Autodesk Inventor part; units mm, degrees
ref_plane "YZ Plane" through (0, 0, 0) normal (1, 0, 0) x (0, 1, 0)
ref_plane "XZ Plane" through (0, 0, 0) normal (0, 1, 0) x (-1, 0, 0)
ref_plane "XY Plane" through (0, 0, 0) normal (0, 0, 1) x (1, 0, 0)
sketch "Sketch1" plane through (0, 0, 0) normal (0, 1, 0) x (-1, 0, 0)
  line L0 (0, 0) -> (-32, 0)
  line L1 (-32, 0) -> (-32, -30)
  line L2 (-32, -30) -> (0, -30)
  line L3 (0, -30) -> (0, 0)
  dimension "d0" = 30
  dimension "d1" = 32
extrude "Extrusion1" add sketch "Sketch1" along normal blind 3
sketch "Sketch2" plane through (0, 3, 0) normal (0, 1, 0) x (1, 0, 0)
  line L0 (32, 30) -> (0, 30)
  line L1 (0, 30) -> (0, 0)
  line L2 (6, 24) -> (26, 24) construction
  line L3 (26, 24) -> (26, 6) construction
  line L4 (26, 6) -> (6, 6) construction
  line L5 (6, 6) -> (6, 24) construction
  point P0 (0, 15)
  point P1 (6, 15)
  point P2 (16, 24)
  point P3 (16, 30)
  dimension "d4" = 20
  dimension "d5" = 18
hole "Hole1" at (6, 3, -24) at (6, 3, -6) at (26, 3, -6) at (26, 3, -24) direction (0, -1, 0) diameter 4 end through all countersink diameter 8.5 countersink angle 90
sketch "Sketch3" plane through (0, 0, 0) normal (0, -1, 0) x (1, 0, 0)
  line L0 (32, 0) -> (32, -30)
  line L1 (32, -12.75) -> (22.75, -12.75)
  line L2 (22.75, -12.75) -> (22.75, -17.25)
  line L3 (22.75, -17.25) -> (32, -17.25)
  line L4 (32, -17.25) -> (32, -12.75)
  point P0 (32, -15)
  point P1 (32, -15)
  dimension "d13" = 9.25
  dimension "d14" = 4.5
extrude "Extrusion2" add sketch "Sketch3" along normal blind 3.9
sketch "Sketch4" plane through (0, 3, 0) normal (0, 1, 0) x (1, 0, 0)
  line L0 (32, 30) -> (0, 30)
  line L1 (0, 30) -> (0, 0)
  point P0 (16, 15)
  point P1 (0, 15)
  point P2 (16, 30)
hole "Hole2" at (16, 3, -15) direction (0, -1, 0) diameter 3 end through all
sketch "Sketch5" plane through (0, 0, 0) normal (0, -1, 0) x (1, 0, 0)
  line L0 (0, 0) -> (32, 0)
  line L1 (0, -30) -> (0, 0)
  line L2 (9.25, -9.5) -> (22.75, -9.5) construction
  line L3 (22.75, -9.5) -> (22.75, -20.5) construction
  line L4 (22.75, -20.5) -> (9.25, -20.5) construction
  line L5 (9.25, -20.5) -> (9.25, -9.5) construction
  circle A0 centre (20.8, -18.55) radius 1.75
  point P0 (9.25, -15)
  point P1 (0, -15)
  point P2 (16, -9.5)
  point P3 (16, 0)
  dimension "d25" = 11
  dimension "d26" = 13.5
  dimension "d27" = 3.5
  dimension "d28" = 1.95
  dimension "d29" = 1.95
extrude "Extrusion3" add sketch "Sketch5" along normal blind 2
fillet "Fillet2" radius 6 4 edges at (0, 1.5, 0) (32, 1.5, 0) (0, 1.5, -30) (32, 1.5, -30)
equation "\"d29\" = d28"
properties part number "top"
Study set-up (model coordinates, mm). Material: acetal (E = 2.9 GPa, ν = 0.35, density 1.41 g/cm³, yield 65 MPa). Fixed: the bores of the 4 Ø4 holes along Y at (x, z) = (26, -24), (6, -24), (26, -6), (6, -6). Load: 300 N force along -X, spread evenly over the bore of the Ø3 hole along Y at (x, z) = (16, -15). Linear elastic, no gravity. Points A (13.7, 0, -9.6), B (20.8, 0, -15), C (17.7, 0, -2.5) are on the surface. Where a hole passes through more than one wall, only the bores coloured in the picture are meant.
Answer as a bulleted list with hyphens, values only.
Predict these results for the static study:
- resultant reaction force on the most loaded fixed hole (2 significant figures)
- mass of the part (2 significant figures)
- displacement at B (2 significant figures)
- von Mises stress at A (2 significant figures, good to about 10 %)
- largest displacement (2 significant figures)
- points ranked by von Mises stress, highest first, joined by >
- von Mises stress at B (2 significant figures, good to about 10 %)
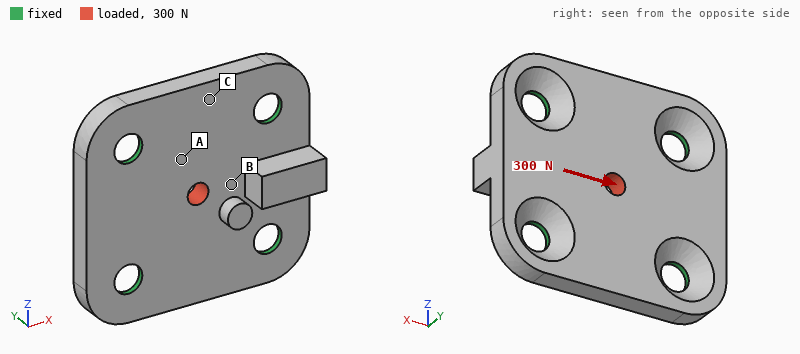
- 80 N
- 3.7 g
- 20 µm
- 3.5 MPa
- 30 µm
- B > A > C
- 6.8 MPa
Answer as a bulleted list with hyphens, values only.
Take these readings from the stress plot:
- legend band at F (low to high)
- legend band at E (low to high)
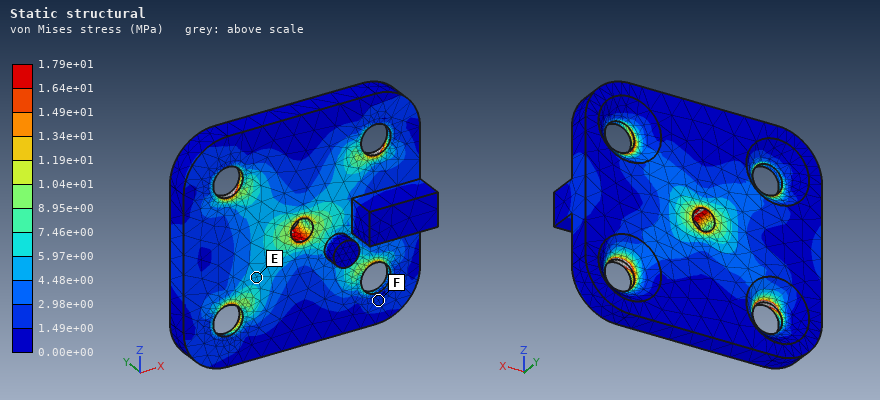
- 1.49e+00 to 2.98e+00 MPa
- 4.48e+00 to 5.97e+00 MPa
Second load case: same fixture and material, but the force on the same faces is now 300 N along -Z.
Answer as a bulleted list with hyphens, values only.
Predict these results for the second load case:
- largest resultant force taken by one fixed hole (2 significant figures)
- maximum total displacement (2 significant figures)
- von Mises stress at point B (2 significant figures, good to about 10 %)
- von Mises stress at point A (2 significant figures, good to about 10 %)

- 81 N
- 32 µm
- 3.2 MPa
- 5.1 MPa
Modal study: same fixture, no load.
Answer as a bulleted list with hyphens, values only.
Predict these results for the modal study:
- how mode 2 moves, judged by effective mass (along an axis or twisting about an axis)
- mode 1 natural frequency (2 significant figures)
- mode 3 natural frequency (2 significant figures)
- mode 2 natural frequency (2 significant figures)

- along Y
- 6900 Hz
- 7900 Hz
- 7500 Hz
